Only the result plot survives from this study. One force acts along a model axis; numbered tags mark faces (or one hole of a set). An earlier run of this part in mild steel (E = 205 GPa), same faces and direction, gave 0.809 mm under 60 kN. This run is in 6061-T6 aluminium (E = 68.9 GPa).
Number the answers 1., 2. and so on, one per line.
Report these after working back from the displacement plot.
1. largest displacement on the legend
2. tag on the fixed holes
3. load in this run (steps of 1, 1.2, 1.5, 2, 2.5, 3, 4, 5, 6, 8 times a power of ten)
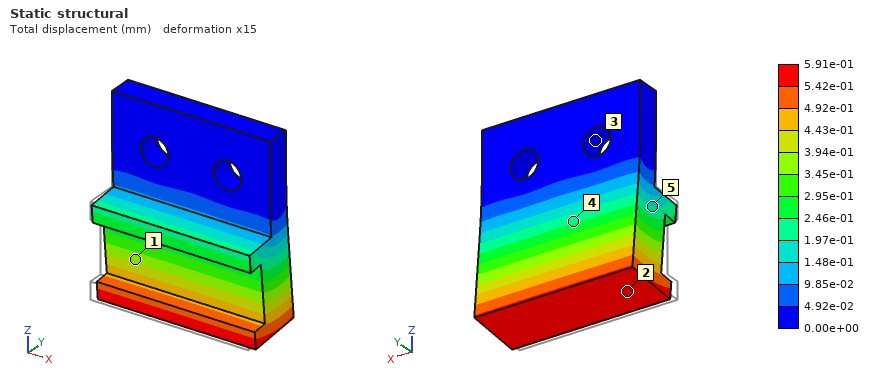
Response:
1. 5.91e-01 mm
2. 3
3. 15 kN
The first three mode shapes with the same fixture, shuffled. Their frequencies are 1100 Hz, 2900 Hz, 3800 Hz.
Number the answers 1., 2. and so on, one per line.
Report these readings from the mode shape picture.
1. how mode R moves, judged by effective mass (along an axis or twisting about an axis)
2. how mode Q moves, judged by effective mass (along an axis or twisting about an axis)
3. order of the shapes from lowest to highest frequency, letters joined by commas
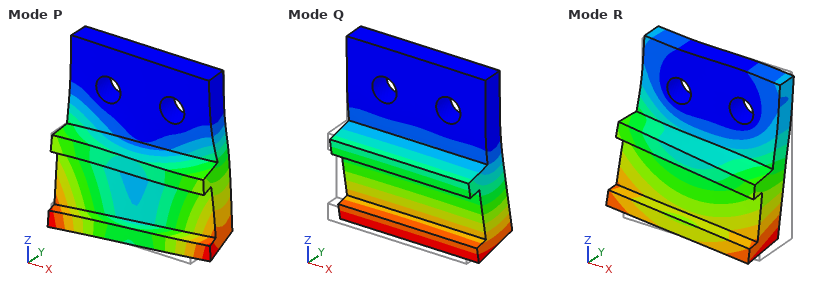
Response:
1. along X
2. along Y
3. Q, P, R
